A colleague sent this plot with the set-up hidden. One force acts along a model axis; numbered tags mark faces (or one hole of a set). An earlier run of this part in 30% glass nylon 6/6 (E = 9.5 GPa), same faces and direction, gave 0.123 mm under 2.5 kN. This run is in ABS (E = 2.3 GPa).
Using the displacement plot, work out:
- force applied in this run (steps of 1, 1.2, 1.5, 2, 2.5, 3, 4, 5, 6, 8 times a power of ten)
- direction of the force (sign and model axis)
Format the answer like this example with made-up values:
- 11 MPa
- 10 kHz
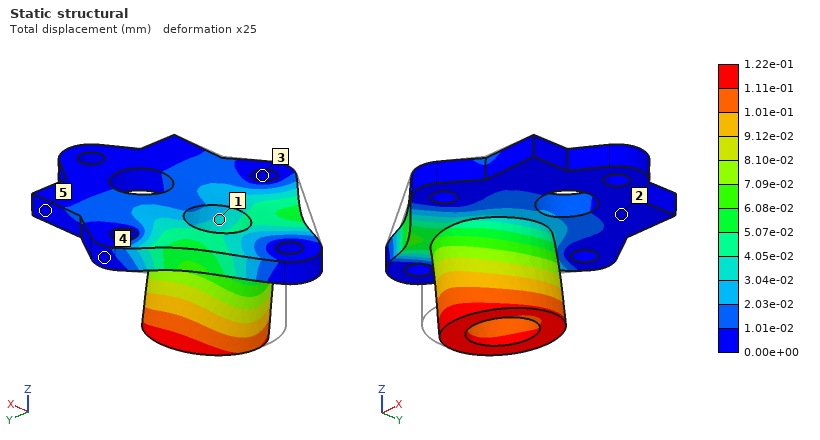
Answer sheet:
- 600 N
- +Y
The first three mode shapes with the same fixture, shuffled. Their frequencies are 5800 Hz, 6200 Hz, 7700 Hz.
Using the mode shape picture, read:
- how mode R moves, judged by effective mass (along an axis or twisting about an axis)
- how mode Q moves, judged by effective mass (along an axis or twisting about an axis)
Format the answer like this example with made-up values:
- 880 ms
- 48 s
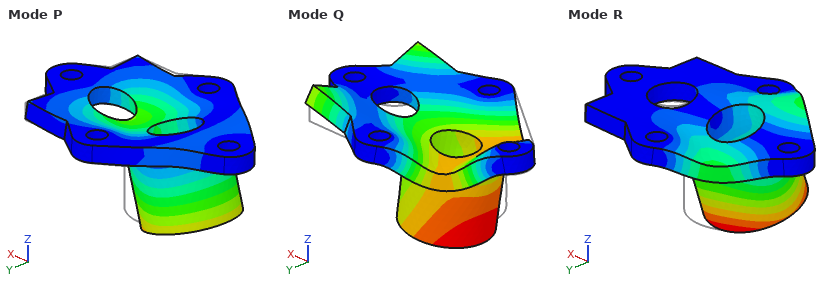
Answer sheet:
- along Y
- along Z
